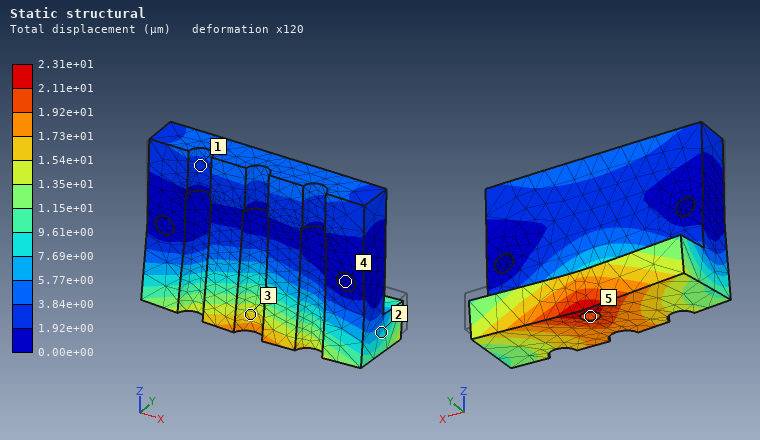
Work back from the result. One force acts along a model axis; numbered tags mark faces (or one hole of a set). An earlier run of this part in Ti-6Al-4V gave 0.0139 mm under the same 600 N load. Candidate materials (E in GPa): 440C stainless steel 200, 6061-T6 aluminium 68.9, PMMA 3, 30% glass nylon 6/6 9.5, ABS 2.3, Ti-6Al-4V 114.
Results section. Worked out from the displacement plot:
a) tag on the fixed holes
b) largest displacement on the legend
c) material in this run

4
2.31e+01 µm
6061-T6 aluminium
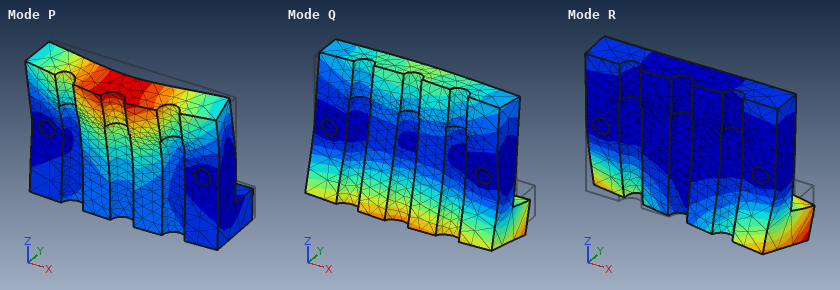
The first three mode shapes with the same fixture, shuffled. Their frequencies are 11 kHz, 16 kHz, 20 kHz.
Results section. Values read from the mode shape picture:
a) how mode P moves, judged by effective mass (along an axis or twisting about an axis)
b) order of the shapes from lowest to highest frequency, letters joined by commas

along Y
Q, P, R
